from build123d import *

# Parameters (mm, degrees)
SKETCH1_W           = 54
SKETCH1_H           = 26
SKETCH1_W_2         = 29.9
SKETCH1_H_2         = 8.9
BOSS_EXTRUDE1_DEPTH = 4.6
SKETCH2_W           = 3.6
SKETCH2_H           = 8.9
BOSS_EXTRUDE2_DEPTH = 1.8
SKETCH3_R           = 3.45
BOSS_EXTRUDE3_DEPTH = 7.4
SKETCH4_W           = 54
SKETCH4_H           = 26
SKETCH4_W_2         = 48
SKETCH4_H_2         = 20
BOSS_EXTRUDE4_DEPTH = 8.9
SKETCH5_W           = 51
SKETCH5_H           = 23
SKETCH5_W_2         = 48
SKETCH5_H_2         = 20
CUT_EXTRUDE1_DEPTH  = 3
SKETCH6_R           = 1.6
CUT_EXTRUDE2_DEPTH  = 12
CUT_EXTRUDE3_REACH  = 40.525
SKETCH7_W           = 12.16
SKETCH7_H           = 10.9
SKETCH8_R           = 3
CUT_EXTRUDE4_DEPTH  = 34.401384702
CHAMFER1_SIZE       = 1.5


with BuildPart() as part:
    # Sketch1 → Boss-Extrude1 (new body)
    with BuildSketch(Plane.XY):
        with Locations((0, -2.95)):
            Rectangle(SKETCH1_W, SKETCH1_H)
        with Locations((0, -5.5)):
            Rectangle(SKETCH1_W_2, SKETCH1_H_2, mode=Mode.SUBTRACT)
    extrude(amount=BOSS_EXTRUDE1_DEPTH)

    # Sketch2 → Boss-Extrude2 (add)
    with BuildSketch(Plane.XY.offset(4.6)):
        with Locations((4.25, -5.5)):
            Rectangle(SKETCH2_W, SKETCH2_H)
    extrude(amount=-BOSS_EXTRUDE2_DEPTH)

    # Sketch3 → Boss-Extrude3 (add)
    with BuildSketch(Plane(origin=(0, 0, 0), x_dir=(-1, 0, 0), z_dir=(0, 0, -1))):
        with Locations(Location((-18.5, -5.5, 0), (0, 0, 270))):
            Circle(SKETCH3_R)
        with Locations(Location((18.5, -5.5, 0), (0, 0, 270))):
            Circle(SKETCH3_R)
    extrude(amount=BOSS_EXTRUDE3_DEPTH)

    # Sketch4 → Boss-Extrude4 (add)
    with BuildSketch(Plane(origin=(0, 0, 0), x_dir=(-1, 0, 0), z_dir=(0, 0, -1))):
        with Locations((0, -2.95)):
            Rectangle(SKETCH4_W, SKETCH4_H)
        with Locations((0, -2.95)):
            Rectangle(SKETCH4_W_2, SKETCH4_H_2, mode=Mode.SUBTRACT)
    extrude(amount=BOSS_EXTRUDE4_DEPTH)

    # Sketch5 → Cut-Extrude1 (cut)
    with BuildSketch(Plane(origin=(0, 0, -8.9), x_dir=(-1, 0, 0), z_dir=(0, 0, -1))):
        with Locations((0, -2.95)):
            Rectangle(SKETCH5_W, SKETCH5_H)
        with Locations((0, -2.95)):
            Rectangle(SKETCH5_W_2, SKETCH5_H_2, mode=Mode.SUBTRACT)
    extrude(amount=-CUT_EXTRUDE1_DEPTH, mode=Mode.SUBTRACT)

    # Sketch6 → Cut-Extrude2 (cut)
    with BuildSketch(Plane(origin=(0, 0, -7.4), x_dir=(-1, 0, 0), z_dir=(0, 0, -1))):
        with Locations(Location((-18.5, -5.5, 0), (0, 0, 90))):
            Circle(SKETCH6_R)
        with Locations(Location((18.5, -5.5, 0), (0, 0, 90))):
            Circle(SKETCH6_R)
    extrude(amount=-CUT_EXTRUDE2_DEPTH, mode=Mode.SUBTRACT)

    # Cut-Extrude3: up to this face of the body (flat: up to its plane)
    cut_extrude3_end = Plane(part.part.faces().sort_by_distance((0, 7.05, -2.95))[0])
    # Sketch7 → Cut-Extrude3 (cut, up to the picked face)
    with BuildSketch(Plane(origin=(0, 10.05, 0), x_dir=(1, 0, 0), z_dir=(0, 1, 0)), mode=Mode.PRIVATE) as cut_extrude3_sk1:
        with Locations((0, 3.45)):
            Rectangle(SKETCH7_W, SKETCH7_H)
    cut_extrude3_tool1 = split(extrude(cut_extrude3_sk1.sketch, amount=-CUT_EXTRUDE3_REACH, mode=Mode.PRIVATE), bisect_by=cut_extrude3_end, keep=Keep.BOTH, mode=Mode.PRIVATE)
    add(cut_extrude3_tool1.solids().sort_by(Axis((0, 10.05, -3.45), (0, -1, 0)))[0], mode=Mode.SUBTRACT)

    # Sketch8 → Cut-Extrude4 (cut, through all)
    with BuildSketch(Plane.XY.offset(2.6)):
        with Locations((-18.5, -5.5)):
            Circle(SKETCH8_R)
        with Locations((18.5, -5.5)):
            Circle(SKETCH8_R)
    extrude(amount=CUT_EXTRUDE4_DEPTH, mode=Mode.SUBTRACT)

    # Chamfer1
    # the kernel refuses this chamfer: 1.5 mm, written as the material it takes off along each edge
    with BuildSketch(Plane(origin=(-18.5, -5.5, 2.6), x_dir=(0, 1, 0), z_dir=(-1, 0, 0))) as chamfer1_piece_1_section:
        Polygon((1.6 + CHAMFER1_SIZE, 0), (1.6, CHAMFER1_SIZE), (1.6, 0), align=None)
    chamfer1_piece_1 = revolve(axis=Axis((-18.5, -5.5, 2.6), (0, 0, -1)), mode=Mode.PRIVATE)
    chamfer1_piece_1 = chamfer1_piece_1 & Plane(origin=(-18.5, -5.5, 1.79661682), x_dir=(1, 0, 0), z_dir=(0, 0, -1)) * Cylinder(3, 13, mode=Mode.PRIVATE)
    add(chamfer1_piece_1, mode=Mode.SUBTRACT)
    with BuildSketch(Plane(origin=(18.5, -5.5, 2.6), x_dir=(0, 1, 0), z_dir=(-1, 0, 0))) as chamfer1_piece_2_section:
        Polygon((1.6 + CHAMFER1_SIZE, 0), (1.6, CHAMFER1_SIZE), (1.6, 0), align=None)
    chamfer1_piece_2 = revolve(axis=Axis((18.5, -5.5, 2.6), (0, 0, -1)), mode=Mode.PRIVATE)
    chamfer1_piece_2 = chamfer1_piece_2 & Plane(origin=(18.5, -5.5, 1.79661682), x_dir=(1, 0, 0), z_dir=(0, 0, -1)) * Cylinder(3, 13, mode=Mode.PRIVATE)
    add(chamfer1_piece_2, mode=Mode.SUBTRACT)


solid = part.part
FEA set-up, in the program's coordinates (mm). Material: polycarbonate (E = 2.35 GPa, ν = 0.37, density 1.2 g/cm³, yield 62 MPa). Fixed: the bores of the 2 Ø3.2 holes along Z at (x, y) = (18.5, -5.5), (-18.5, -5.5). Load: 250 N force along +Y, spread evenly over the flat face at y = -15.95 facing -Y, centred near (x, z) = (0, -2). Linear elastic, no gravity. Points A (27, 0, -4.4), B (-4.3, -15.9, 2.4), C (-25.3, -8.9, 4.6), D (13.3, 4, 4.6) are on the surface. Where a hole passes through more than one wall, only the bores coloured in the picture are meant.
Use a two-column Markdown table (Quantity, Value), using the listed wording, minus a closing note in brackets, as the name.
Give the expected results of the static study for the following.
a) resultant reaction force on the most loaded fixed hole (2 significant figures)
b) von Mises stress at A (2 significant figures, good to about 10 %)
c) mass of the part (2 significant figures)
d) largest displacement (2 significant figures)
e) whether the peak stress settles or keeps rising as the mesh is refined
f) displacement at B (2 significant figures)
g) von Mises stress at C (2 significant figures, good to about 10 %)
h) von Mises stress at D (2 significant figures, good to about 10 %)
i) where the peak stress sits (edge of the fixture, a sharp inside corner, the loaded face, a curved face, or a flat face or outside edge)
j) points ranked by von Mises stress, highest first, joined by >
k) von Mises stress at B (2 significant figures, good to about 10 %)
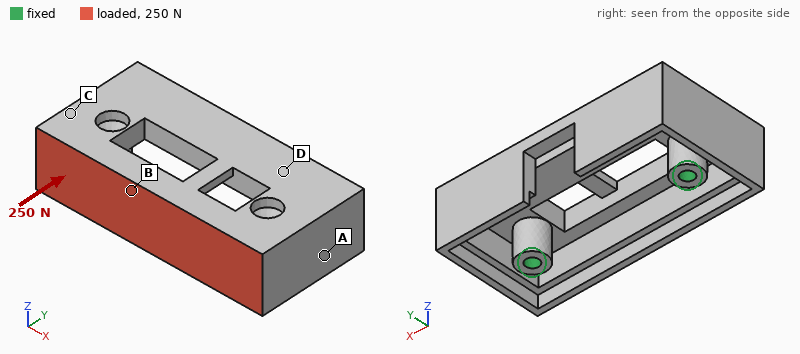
| Quantity | Value |
|---|---|
| resultant reaction force on the most loaded fixed hole | 130 N |
| von Mises stress at A | 1.3 MPa |
| mass of the part | 10 g |
| largest displacement | 0.53 mm |
| whether the peak stress settles or keeps rising as the mesh is refined | keeps rising |
| displacement at B | 0.17 mm |
| von Mises stress at C | 4.6 MPa |
| von Mises stress at D | 2.4 MPa |
| where the peak stress sits | a sharp inside corner |
| points ranked by von Mises stress, highest first, joined by > | B > C > D > A |
| von Mises stress at B | 6.7 MPa |
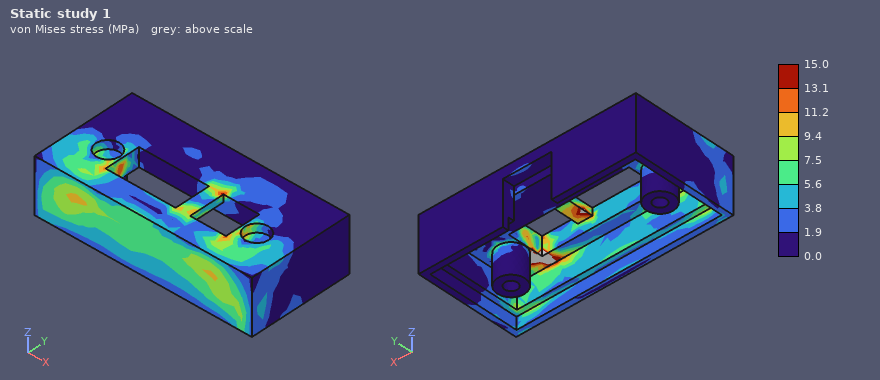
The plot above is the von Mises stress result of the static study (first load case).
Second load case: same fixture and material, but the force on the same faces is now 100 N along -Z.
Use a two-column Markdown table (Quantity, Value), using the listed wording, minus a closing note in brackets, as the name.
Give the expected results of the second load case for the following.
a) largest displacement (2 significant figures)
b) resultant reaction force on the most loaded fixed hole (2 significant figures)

| Quantity | Value |
|---|---|
| largest displacement | 0.28 mm |
| resultant reaction force on the most loaded fixed hole | 50 N |
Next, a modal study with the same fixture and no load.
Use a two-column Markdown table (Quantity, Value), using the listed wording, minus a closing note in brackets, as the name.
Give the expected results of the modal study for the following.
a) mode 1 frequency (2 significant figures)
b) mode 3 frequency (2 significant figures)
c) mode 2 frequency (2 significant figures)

| Quantity | Value |
|---|---|
| mode 1 frequency | 1500 Hz |
| mode 3 frequency | 2400 Hz |
| mode 2 frequency | 2200 Hz |
